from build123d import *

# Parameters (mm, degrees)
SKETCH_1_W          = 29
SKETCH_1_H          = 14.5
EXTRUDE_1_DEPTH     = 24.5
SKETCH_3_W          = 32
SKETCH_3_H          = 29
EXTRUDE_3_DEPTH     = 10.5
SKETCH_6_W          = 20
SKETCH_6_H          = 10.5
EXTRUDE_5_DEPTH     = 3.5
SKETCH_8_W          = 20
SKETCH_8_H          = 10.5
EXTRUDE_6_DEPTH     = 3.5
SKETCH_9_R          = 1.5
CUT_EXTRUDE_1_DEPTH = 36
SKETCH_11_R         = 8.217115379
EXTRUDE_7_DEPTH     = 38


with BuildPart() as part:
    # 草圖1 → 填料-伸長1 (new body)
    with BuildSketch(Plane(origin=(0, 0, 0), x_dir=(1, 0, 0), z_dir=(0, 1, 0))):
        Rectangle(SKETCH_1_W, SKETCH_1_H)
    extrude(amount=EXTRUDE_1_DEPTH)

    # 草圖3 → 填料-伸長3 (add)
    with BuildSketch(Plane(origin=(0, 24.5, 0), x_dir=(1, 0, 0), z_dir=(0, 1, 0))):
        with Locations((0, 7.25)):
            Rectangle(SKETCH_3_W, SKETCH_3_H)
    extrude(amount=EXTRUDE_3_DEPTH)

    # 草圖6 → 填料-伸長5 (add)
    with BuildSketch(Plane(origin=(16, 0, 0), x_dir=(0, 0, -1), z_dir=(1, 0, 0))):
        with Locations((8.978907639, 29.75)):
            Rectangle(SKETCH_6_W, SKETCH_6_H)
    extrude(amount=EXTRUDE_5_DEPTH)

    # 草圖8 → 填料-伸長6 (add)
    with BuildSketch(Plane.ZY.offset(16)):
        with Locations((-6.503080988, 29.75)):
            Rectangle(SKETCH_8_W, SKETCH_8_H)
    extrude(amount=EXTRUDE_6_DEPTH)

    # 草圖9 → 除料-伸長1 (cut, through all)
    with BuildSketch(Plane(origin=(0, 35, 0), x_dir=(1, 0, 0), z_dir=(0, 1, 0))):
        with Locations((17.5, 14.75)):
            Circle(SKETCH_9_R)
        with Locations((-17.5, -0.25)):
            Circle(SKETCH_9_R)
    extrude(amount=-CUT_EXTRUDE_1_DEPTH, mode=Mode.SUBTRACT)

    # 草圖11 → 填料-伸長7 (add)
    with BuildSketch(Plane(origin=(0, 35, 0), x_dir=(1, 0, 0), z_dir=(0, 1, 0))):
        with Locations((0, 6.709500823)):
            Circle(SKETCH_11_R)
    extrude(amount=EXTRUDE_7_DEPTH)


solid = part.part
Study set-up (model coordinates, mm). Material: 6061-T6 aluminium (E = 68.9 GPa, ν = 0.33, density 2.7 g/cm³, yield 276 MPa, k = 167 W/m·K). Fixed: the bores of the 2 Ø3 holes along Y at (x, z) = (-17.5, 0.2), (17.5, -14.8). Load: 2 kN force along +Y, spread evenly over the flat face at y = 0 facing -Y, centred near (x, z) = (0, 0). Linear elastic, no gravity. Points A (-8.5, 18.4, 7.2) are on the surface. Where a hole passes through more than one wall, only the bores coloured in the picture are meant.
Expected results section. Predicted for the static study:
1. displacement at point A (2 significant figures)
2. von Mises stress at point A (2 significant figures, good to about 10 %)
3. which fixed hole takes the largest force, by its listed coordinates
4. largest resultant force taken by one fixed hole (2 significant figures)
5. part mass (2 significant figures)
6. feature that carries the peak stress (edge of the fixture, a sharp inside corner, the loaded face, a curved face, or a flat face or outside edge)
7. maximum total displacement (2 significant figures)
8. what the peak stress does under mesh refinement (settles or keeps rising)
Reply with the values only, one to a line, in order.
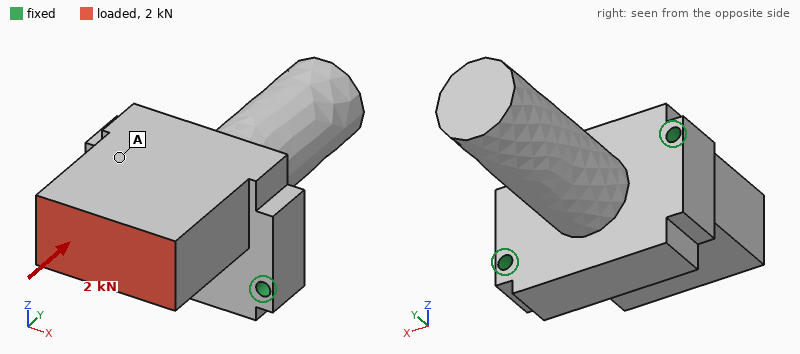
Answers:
12 µm
7.6 MPa
(-17.5, 0.2)
1.1 kN
79 g
edge of the fixture
29 µm
keeps rising
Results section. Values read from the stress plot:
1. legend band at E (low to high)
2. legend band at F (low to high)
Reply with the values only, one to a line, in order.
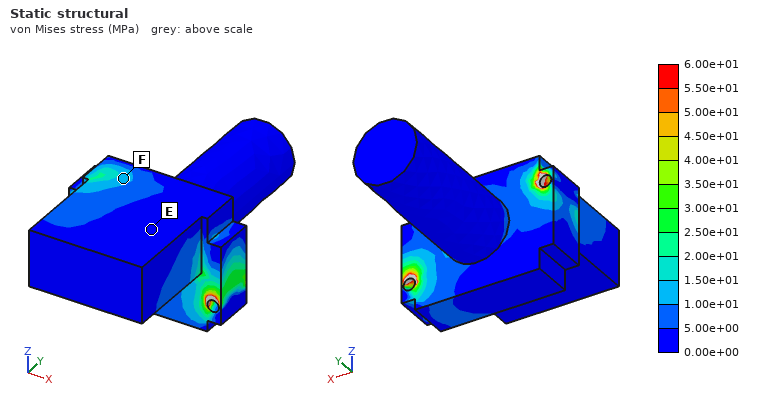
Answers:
0.00e+00 to 5.00e+00 MPa
1.00e+01 to 1.50e+01 MPa
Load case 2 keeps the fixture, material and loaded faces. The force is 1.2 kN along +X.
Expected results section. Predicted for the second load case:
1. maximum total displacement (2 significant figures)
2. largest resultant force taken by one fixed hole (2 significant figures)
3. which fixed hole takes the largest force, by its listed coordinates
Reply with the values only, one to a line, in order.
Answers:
36 µm
1.3 kN
(-17.5, 0.2)
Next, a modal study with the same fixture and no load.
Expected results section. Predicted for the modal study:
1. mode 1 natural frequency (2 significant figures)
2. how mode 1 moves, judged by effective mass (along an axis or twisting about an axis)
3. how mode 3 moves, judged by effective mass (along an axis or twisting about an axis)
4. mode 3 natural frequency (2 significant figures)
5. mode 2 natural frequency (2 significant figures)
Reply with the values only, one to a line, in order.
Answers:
3700 Hz
twisting about X
along Z
7800 Hz
5900 Hz
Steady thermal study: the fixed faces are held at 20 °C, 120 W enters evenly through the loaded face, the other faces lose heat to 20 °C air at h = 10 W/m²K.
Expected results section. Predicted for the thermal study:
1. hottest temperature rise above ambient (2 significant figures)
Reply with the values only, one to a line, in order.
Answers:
70 K
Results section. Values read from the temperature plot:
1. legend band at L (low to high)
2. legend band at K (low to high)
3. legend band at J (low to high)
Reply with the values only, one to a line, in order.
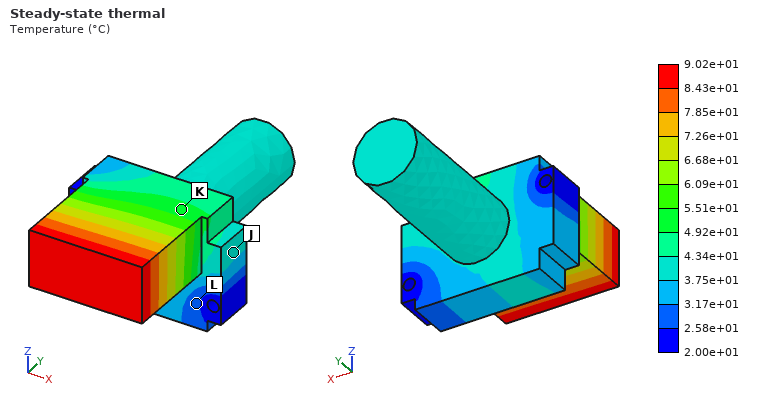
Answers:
2.58e+01 to 3.17e+01 °C
4.92e+01 to 5.51e+01 °C
3.75e+01 to 4.34e+01 °C
